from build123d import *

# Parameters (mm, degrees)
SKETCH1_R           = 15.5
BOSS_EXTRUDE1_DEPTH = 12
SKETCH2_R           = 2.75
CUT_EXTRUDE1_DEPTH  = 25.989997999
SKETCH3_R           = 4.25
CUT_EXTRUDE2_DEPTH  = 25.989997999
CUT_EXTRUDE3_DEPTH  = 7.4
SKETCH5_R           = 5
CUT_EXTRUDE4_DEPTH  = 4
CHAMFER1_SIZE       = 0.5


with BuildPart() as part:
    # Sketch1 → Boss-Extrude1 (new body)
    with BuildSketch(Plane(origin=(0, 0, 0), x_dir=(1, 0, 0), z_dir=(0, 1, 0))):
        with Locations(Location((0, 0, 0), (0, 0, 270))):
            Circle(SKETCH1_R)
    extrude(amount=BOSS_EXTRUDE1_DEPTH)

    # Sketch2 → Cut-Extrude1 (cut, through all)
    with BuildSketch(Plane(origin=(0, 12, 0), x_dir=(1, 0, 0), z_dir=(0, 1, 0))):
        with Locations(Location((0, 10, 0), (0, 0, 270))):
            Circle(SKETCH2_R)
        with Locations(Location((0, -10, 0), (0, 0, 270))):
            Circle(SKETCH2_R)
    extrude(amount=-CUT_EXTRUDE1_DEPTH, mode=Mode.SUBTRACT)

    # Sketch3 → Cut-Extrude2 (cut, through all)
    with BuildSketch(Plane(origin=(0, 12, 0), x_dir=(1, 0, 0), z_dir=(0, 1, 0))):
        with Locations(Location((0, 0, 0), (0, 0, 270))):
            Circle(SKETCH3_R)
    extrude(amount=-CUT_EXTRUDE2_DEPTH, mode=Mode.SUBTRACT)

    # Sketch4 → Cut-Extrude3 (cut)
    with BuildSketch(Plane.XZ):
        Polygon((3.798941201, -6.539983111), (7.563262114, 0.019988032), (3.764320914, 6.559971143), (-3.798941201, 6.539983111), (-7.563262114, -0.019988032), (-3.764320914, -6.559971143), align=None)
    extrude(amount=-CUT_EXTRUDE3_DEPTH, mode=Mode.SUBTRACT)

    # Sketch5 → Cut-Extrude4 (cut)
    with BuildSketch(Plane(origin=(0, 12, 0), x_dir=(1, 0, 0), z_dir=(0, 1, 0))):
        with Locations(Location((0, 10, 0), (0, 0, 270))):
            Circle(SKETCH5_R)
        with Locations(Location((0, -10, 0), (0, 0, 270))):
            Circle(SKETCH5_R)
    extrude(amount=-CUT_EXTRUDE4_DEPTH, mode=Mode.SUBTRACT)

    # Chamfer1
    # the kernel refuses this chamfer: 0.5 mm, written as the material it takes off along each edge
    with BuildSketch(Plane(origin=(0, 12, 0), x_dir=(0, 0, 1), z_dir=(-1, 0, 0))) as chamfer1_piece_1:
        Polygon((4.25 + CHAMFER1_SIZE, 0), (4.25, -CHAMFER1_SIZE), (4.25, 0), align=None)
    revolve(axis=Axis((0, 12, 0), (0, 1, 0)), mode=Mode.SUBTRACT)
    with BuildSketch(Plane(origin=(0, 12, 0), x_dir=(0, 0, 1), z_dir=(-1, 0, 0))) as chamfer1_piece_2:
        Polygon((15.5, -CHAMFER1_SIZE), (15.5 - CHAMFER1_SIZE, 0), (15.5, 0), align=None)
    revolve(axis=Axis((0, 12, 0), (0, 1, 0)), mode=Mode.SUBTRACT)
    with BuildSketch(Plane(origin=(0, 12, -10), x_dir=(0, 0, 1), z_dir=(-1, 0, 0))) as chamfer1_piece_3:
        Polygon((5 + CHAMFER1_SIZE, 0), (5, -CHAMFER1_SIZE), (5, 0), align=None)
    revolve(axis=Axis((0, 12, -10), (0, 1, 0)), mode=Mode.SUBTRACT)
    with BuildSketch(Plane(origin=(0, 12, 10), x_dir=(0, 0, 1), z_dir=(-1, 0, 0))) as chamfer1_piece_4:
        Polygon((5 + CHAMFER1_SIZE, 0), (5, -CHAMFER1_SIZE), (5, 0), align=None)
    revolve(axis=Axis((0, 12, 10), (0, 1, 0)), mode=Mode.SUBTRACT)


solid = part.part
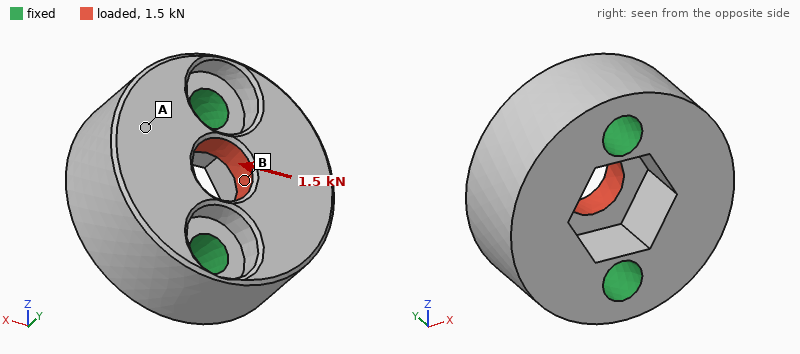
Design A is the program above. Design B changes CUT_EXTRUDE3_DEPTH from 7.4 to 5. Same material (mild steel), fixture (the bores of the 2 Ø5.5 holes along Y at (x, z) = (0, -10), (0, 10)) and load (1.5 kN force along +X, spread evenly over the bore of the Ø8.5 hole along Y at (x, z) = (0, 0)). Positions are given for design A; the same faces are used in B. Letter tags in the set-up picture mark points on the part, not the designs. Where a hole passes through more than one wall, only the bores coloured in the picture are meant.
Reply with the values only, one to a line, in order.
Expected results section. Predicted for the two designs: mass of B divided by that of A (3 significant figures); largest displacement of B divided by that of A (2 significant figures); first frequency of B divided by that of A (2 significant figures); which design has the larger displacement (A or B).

1.03
0.67
1.0
A
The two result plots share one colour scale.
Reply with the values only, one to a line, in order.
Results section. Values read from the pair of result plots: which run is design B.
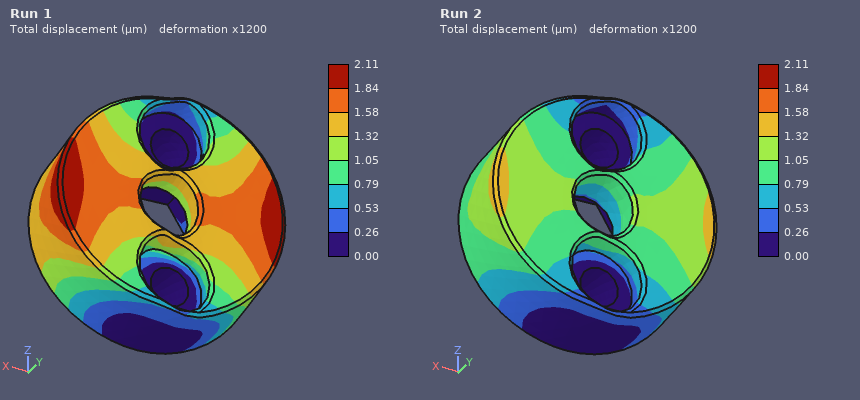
Run 2
